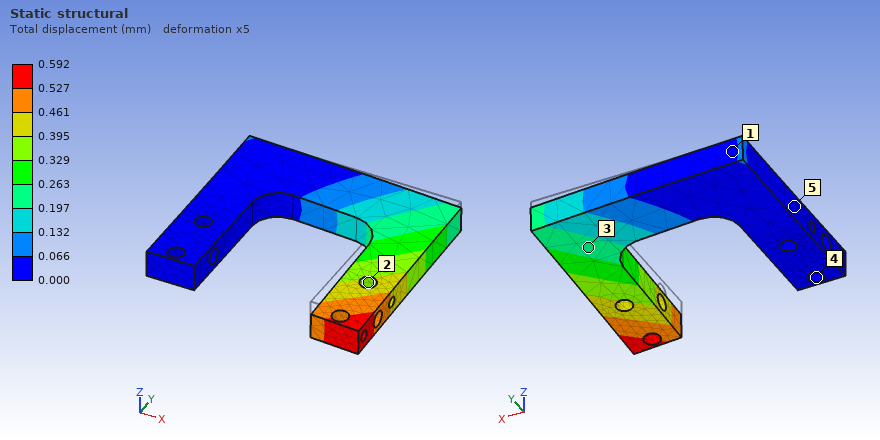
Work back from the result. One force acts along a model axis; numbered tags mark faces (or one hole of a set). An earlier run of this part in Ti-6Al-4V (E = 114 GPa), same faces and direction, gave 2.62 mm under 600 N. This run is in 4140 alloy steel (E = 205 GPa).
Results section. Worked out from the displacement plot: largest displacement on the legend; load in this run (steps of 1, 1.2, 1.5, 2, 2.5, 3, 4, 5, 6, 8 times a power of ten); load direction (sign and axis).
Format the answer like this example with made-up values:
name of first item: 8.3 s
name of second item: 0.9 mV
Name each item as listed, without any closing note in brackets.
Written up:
largest displacement on the legend: 0.592 mm
load in this run: 250 N
load direction: -Z
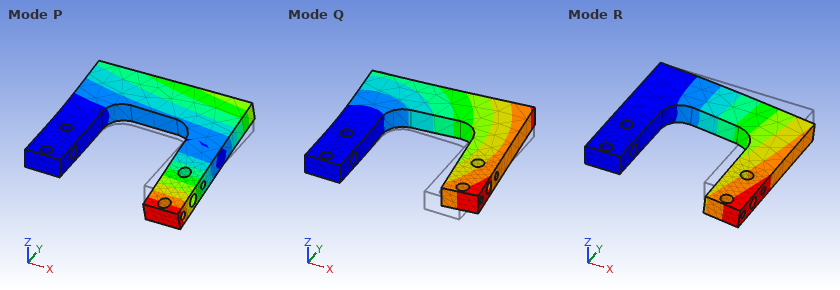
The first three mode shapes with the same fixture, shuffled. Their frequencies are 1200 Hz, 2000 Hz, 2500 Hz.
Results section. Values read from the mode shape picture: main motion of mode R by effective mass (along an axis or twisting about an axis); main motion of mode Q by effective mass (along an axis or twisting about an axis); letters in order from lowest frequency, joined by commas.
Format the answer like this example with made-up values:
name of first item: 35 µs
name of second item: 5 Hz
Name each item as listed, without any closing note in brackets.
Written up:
main motion of mode R by effective mass: along Z
main motion of mode Q by effective mass: along Y
letters in order from lowest frequency, joined by commas: R, Q, P
